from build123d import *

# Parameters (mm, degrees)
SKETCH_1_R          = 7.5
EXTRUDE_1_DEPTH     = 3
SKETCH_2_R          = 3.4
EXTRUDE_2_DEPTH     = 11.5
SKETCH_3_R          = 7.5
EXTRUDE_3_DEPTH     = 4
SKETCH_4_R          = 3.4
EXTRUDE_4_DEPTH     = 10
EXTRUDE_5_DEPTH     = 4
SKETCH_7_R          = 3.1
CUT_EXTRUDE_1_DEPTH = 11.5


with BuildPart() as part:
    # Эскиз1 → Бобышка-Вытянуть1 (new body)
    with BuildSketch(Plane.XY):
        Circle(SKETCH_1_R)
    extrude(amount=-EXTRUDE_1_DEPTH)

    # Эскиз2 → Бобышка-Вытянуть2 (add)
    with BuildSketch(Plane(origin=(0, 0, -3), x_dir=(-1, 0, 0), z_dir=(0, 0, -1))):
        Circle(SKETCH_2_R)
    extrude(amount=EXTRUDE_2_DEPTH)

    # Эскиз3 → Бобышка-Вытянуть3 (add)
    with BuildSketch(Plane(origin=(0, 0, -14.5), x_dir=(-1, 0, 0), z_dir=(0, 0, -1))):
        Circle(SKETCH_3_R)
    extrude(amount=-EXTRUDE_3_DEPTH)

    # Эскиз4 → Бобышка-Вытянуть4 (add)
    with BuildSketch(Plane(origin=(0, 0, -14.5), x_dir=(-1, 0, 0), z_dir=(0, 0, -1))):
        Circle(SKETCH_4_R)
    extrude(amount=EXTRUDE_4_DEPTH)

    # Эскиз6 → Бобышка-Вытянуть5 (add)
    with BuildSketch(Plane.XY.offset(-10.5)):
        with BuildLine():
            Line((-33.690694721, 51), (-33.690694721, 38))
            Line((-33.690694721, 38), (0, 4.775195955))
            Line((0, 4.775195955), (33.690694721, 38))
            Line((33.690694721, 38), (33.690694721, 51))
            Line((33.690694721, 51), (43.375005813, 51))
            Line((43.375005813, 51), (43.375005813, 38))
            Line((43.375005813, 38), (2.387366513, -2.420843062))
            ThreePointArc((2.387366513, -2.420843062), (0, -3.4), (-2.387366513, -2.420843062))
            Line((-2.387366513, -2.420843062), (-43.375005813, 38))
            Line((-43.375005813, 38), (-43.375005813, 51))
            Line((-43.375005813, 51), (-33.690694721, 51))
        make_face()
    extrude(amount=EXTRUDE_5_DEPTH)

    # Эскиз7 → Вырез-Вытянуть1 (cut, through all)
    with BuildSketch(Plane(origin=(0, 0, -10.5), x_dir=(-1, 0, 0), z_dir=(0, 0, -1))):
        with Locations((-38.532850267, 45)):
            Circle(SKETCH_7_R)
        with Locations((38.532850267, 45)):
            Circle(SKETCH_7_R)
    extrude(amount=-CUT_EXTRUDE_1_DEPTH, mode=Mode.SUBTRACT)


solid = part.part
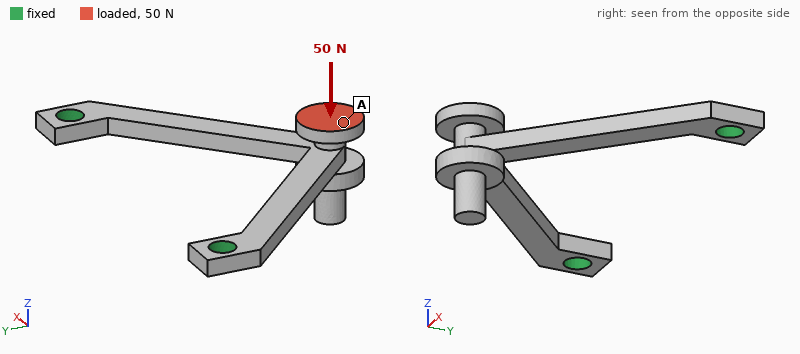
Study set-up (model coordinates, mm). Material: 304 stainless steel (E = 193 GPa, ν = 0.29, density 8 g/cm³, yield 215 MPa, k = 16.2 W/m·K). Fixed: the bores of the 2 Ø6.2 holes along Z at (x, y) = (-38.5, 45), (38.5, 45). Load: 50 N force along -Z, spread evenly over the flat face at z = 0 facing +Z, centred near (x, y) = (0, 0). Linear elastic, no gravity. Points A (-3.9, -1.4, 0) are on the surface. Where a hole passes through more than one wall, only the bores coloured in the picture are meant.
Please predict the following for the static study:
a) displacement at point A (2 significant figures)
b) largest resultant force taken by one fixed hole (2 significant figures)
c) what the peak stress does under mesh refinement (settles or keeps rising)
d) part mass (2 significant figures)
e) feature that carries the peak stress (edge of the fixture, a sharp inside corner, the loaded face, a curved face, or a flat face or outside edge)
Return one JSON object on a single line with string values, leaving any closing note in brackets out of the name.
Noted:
{"displacement at point A": "0.14 mm", "largest resultant force taken by one fixed hole": "25 N", "what the peak stress does under mesh refinement": "keeps rising", "part mass": "43 g", "feature that carries the peak stress": "a sharp inside corner"}
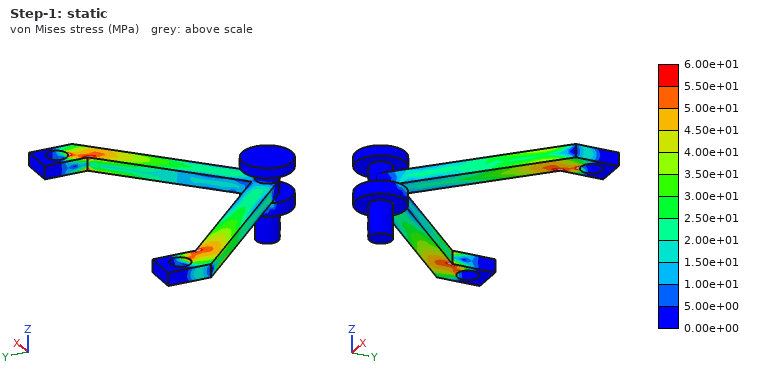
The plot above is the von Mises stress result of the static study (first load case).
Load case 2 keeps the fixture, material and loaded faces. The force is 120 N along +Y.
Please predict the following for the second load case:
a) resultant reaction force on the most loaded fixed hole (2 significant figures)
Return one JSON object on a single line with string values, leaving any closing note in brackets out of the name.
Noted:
{"resultant reaction force on the most loaded fixed hole": "82 N"}
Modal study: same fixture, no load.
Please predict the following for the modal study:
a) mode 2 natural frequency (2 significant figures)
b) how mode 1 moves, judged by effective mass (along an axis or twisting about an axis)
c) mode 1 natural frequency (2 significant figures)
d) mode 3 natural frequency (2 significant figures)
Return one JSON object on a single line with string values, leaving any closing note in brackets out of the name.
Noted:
{"mode 2 natural frequency": "3500 Hz", "how mode 1 moves, judged by effective mass": "along Z", "mode 1 natural frequency": "680 Hz", "mode 3 natural frequency": "3600 Hz"}
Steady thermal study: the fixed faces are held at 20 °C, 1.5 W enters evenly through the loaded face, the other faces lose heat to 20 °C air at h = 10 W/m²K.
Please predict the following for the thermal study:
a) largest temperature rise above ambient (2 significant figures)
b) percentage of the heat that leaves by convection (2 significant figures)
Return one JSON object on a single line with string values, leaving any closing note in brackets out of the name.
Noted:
{"largest temperature rise above ambient": "60 K", "percentage of the heat that leaves by convection": "62 %"}
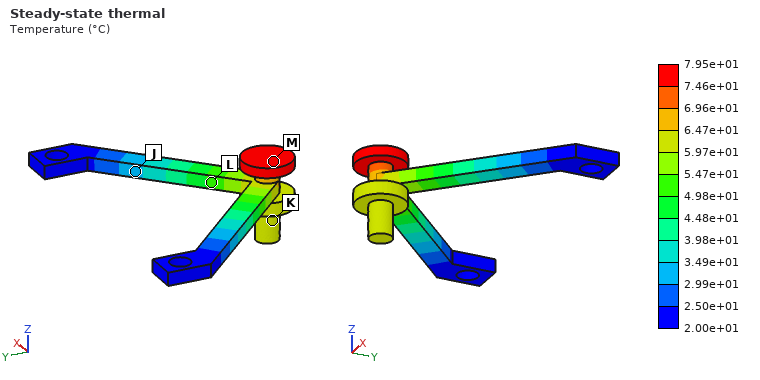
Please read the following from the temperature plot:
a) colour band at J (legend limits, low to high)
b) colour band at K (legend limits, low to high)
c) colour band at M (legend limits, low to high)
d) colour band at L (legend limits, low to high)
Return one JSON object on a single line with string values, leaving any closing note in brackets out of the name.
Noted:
{"colour band at J": "2.99e+01 to 3.49e+01 °C", "colour band at K": "5.97e+01 to 6.47e+01 °C", "colour band at M": "7.46e+01 to 7.95e+01 °C", "colour band at L": "4.98e+01 to 5.47e+01 °C"}
